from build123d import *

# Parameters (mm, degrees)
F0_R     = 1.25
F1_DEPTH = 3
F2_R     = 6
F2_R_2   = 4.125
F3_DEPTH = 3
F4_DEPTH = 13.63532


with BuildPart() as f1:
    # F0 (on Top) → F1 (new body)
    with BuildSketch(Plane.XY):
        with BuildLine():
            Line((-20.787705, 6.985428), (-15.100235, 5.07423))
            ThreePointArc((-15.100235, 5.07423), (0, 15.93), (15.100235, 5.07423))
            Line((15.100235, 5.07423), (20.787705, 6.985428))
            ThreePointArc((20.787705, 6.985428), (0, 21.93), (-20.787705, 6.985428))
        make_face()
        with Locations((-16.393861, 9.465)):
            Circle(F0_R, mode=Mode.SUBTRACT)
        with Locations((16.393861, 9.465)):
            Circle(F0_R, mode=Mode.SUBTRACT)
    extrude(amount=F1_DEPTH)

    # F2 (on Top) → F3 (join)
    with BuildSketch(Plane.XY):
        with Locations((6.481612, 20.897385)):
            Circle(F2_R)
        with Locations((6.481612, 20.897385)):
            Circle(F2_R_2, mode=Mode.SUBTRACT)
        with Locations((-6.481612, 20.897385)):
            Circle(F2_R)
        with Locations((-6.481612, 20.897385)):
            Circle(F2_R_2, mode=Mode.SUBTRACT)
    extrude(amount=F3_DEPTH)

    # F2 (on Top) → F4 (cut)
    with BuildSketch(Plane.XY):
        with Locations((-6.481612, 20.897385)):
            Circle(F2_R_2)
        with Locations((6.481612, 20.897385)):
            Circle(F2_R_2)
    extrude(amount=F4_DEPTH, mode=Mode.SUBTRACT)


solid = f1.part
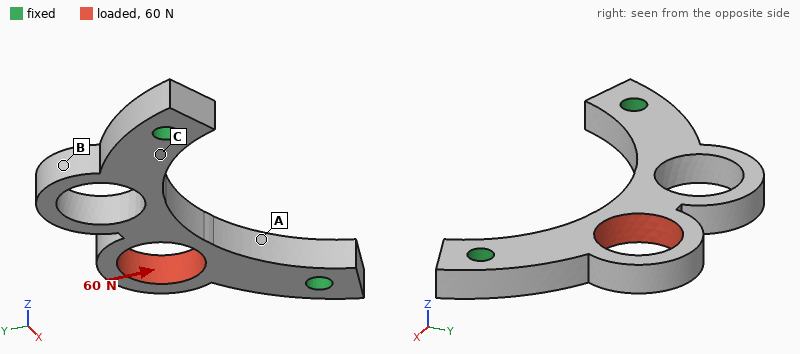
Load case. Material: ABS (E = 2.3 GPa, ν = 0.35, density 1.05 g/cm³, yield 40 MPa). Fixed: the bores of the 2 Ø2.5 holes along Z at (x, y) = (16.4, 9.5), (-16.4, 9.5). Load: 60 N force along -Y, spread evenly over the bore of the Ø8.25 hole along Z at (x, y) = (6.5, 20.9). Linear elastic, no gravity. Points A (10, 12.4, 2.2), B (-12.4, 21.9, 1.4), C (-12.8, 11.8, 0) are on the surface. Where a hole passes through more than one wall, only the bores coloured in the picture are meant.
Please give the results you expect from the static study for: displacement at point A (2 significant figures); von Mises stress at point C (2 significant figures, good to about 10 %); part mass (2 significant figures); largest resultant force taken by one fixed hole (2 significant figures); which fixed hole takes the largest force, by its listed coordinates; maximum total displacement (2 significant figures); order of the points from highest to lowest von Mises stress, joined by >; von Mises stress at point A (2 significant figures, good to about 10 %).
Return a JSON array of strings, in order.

["35 µm", "3.2 MPa", "0.90 g", "54 N", "(16.4, 9.5)", "85 µm", "A > C > B", "6.3 MPa"]
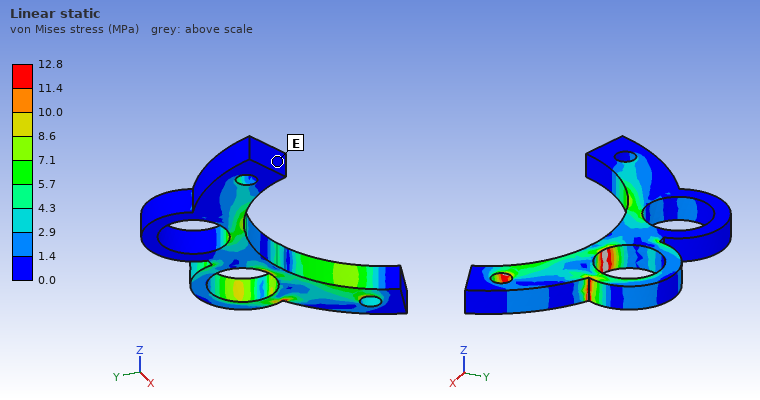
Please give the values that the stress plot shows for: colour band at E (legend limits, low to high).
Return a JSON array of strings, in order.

["0.0 to 1.4 MPa"]
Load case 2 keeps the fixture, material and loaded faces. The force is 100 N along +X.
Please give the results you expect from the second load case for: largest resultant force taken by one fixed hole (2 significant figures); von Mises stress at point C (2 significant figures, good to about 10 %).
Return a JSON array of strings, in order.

["59 N", "5.2 MPa"]
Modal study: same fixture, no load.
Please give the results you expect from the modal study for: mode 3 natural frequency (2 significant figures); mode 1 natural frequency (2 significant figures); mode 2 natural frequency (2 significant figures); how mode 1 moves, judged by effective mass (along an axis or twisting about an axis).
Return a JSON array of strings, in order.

["5700 Hz", "1800 Hz", "4200 Hz", "along Z"]
